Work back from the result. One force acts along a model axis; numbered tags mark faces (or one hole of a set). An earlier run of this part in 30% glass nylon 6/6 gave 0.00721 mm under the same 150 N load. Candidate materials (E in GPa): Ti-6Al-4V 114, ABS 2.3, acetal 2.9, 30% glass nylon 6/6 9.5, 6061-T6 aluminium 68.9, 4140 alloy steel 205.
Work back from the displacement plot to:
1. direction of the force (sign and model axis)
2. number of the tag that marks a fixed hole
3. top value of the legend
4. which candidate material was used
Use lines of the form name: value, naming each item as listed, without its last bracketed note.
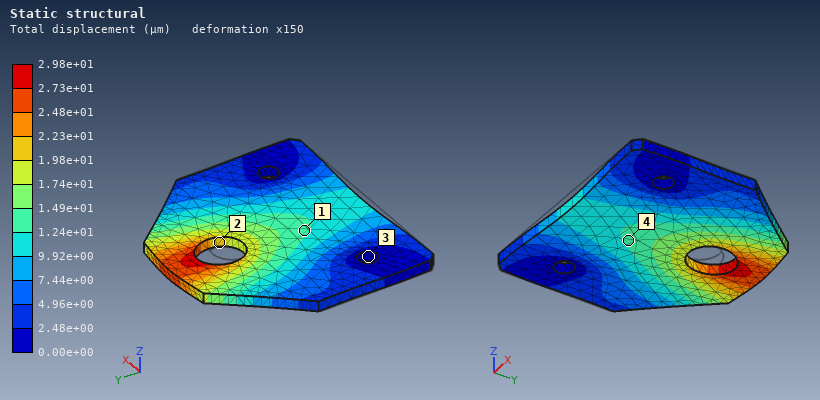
direction of the force: +Y
number of the tag that marks a fixed hole: 3
top value of the legend: 2.98e+01 µm
which candidate material was used: ABS
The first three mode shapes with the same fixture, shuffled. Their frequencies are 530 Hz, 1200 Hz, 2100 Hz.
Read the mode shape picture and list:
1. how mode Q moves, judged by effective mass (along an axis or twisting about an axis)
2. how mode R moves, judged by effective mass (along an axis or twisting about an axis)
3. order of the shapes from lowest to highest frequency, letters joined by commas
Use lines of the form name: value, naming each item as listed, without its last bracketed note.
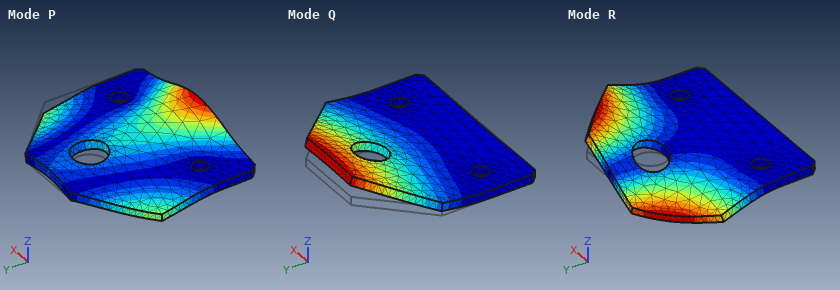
how mode Q moves, judged by effective mass: along Z
how mode R moves, judged by effective mass: twisting about Y
order of the shapes from lowest to highest frequency, letters joined by commas: Q, R, P
